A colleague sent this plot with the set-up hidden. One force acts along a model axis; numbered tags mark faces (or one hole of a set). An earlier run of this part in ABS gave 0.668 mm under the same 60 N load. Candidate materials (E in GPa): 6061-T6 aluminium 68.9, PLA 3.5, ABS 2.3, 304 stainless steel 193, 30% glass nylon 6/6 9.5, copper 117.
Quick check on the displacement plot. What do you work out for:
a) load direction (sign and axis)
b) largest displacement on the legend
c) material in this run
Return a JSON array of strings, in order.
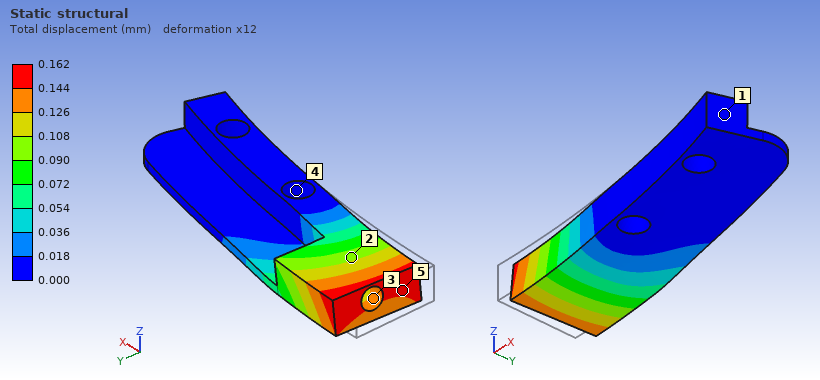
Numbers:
["+Y", "0.162 mm", "30% glass nylon 6/6"]
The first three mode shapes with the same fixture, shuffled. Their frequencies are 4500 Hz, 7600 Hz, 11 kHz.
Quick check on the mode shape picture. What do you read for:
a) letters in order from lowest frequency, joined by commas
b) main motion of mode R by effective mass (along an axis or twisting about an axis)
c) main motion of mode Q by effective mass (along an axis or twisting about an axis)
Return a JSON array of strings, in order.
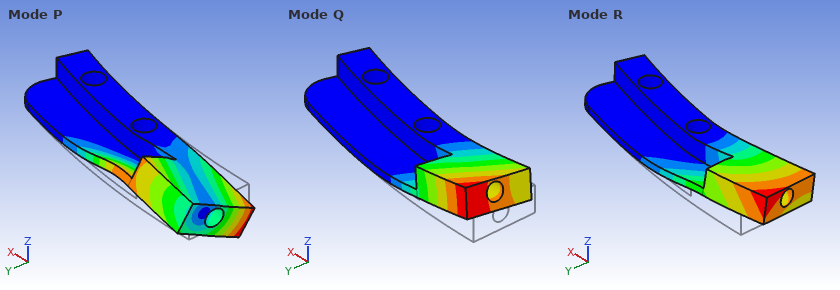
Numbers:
["Q, R, P", "along Y", "along Z"]
